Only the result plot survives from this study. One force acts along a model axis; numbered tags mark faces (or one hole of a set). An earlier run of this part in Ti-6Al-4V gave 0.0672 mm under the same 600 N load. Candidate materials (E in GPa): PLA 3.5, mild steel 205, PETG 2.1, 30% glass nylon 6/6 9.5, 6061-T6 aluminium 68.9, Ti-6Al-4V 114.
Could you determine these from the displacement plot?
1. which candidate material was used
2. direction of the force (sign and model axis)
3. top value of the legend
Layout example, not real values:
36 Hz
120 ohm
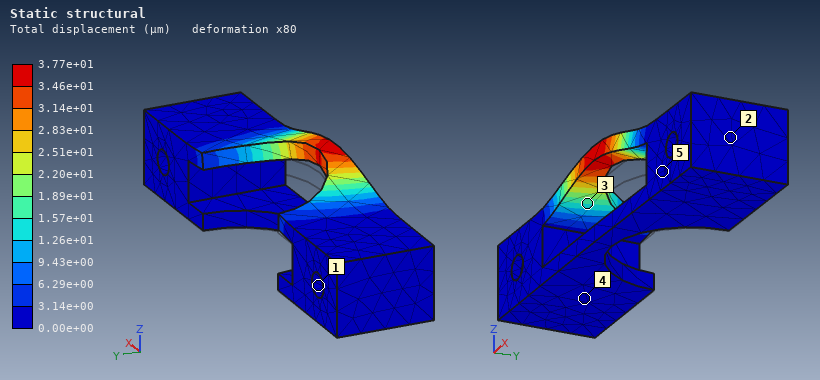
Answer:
mild steel
+Z
3.77e+01 µm
